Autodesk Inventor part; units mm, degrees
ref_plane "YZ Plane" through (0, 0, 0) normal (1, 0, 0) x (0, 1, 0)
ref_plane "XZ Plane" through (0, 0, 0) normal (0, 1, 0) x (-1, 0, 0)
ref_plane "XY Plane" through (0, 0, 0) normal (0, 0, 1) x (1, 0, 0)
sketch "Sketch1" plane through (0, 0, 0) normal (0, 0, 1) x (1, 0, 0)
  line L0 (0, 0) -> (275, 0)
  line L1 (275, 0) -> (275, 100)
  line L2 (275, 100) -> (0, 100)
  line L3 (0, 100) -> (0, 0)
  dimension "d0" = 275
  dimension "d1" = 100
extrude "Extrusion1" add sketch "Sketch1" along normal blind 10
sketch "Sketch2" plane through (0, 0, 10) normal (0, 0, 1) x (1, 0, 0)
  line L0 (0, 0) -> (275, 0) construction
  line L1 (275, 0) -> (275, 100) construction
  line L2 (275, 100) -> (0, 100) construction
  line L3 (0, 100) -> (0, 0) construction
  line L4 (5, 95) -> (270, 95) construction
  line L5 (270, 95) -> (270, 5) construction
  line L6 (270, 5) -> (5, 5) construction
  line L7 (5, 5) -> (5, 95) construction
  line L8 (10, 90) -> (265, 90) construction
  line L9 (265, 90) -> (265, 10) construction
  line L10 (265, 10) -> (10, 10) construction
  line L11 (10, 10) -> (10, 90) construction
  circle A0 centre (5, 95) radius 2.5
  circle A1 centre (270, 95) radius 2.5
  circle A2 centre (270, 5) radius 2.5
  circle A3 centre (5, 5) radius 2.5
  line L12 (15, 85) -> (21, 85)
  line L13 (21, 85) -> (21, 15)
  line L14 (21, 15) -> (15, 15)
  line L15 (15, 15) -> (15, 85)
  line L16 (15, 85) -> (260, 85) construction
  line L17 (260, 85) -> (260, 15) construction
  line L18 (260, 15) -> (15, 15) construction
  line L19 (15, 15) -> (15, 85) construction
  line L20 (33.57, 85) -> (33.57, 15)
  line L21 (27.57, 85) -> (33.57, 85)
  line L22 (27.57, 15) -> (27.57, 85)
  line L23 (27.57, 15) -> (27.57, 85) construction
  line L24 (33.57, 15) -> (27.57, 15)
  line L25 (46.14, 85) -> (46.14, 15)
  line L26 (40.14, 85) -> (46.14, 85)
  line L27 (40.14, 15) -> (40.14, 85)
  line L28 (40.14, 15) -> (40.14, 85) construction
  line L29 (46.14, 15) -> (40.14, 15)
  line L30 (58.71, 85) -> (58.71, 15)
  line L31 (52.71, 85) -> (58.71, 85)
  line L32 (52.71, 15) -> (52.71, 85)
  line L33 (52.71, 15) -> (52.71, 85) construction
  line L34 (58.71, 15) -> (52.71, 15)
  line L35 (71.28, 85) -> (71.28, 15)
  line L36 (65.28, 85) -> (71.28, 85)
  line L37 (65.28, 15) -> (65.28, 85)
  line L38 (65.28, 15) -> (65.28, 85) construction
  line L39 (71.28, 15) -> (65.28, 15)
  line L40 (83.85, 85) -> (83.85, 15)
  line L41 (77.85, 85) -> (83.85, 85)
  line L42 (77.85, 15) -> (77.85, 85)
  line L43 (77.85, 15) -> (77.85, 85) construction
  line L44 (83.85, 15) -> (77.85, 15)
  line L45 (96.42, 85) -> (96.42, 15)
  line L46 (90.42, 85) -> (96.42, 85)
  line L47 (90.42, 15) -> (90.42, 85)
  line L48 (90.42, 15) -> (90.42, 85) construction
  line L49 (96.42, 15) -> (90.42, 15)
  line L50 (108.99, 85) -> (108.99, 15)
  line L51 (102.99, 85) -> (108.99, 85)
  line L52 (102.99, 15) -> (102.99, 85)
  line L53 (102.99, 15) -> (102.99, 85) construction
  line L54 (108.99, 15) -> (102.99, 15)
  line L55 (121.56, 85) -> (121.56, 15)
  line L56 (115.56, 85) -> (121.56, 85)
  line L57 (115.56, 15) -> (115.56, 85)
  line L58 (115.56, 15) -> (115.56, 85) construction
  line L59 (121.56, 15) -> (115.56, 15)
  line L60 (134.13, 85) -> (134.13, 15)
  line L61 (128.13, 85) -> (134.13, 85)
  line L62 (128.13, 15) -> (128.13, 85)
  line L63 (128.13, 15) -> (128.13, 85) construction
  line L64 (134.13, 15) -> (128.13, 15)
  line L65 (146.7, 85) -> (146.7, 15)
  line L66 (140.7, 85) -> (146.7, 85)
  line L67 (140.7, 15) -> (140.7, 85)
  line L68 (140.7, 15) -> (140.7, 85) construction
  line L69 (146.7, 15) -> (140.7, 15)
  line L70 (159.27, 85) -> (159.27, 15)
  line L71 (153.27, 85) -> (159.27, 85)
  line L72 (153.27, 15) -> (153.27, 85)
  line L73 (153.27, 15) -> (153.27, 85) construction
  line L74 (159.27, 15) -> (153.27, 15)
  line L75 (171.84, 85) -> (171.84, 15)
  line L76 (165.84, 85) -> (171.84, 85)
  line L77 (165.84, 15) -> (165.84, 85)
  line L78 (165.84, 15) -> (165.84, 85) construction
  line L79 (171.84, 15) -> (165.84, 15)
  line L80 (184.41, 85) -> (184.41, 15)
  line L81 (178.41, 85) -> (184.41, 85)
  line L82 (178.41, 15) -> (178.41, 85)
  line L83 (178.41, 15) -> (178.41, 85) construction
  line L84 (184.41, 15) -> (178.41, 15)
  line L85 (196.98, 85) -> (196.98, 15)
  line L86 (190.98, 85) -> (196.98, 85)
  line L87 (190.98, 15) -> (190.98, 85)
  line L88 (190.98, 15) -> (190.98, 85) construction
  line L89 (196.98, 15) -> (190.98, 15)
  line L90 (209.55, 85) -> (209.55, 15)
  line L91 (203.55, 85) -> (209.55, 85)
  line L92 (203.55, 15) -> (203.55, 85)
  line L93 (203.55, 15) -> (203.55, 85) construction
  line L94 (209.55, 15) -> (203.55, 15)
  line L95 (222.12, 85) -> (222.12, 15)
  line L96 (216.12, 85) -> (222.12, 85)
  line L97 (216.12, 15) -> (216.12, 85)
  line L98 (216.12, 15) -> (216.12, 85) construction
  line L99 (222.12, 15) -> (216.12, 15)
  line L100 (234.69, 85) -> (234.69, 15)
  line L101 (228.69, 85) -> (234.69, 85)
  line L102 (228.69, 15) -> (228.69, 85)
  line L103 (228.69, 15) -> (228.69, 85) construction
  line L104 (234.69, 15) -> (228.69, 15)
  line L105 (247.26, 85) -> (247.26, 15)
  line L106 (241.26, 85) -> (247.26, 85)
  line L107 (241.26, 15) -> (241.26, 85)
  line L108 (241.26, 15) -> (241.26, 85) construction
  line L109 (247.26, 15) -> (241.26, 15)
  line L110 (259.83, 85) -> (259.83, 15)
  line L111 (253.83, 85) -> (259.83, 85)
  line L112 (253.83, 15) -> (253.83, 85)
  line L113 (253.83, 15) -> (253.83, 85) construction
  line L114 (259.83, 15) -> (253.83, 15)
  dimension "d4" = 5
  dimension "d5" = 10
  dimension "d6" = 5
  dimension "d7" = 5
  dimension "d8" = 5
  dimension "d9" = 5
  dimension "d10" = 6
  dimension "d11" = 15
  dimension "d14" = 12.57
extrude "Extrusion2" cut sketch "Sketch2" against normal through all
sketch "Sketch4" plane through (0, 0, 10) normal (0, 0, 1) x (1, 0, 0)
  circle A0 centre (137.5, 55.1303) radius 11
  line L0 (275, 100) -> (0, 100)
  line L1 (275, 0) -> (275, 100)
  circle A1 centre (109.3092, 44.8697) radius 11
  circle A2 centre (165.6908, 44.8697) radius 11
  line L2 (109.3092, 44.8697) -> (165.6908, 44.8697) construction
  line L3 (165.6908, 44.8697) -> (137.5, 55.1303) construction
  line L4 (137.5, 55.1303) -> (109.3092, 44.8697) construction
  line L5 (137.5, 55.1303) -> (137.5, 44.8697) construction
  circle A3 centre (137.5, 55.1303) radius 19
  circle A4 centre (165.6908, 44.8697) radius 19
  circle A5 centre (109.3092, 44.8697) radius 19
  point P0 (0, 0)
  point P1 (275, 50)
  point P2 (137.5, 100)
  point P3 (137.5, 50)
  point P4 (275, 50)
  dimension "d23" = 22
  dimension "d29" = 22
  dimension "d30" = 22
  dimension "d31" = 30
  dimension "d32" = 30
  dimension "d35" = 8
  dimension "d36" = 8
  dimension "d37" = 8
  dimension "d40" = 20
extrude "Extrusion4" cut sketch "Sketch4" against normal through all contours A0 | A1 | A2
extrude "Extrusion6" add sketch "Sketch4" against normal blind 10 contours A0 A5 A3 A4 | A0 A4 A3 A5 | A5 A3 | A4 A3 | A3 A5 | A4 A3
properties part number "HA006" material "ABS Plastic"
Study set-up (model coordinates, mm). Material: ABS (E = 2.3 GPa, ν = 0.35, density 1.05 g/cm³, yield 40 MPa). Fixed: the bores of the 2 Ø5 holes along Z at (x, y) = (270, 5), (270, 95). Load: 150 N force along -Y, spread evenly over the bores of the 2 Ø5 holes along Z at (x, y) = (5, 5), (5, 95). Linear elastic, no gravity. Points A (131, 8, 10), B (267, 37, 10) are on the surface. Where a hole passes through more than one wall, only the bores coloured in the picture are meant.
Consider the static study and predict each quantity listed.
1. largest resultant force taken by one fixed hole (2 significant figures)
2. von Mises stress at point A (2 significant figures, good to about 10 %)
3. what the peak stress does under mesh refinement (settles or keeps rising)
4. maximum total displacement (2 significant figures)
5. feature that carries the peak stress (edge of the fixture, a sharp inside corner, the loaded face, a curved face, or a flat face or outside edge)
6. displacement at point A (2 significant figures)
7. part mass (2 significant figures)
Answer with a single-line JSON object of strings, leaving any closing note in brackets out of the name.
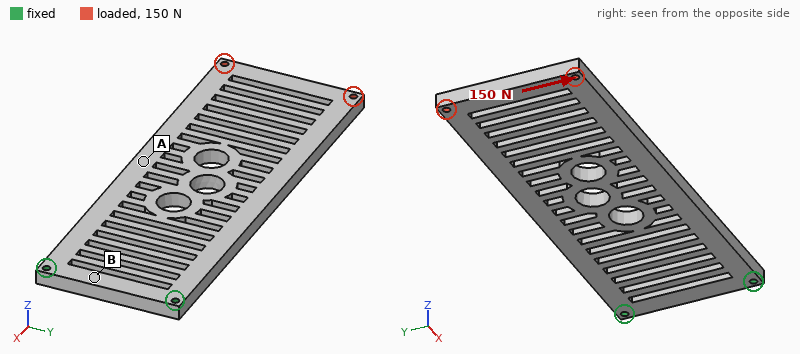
{"largest resultant force taken by one fixed hole": "430 N", "von Mises stress at point A": "1.4 MPa", "what the peak stress does under mesh refinement": "keeps rising", "maximum total displacement": "2.0 mm", "feature that carries the peak stress": "edge of the fixture", "displacement at point A": "0.83 mm", "part mass": "200 g"}
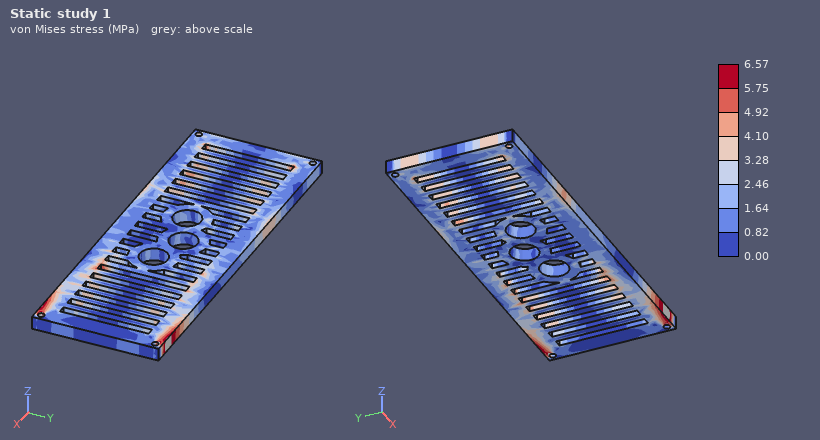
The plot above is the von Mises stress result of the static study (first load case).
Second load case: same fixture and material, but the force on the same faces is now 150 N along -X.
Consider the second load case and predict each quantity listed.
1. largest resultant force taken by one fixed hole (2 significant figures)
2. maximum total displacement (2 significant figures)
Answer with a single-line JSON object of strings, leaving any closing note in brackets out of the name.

{"largest resultant force taken by one fixed hole": "75 N", "maximum total displacement": "59 µm"}
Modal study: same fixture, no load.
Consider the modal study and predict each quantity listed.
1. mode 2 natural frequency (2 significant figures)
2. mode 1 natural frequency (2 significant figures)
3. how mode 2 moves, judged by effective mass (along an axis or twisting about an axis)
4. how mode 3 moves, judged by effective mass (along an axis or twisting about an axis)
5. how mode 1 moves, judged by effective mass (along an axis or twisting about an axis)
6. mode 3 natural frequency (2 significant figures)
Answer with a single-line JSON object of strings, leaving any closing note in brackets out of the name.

{"mode 2 natural frequency": "130 Hz", "mode 1 natural frequency": "22 Hz", "how mode 2 moves, judged by effective mass": "twisting about X", "how mode 3 moves, judged by effective mass": "along Z", "how mode 1 moves, judged by effective mass": "along Z", "mode 3 natural frequency": "140 Hz"}
